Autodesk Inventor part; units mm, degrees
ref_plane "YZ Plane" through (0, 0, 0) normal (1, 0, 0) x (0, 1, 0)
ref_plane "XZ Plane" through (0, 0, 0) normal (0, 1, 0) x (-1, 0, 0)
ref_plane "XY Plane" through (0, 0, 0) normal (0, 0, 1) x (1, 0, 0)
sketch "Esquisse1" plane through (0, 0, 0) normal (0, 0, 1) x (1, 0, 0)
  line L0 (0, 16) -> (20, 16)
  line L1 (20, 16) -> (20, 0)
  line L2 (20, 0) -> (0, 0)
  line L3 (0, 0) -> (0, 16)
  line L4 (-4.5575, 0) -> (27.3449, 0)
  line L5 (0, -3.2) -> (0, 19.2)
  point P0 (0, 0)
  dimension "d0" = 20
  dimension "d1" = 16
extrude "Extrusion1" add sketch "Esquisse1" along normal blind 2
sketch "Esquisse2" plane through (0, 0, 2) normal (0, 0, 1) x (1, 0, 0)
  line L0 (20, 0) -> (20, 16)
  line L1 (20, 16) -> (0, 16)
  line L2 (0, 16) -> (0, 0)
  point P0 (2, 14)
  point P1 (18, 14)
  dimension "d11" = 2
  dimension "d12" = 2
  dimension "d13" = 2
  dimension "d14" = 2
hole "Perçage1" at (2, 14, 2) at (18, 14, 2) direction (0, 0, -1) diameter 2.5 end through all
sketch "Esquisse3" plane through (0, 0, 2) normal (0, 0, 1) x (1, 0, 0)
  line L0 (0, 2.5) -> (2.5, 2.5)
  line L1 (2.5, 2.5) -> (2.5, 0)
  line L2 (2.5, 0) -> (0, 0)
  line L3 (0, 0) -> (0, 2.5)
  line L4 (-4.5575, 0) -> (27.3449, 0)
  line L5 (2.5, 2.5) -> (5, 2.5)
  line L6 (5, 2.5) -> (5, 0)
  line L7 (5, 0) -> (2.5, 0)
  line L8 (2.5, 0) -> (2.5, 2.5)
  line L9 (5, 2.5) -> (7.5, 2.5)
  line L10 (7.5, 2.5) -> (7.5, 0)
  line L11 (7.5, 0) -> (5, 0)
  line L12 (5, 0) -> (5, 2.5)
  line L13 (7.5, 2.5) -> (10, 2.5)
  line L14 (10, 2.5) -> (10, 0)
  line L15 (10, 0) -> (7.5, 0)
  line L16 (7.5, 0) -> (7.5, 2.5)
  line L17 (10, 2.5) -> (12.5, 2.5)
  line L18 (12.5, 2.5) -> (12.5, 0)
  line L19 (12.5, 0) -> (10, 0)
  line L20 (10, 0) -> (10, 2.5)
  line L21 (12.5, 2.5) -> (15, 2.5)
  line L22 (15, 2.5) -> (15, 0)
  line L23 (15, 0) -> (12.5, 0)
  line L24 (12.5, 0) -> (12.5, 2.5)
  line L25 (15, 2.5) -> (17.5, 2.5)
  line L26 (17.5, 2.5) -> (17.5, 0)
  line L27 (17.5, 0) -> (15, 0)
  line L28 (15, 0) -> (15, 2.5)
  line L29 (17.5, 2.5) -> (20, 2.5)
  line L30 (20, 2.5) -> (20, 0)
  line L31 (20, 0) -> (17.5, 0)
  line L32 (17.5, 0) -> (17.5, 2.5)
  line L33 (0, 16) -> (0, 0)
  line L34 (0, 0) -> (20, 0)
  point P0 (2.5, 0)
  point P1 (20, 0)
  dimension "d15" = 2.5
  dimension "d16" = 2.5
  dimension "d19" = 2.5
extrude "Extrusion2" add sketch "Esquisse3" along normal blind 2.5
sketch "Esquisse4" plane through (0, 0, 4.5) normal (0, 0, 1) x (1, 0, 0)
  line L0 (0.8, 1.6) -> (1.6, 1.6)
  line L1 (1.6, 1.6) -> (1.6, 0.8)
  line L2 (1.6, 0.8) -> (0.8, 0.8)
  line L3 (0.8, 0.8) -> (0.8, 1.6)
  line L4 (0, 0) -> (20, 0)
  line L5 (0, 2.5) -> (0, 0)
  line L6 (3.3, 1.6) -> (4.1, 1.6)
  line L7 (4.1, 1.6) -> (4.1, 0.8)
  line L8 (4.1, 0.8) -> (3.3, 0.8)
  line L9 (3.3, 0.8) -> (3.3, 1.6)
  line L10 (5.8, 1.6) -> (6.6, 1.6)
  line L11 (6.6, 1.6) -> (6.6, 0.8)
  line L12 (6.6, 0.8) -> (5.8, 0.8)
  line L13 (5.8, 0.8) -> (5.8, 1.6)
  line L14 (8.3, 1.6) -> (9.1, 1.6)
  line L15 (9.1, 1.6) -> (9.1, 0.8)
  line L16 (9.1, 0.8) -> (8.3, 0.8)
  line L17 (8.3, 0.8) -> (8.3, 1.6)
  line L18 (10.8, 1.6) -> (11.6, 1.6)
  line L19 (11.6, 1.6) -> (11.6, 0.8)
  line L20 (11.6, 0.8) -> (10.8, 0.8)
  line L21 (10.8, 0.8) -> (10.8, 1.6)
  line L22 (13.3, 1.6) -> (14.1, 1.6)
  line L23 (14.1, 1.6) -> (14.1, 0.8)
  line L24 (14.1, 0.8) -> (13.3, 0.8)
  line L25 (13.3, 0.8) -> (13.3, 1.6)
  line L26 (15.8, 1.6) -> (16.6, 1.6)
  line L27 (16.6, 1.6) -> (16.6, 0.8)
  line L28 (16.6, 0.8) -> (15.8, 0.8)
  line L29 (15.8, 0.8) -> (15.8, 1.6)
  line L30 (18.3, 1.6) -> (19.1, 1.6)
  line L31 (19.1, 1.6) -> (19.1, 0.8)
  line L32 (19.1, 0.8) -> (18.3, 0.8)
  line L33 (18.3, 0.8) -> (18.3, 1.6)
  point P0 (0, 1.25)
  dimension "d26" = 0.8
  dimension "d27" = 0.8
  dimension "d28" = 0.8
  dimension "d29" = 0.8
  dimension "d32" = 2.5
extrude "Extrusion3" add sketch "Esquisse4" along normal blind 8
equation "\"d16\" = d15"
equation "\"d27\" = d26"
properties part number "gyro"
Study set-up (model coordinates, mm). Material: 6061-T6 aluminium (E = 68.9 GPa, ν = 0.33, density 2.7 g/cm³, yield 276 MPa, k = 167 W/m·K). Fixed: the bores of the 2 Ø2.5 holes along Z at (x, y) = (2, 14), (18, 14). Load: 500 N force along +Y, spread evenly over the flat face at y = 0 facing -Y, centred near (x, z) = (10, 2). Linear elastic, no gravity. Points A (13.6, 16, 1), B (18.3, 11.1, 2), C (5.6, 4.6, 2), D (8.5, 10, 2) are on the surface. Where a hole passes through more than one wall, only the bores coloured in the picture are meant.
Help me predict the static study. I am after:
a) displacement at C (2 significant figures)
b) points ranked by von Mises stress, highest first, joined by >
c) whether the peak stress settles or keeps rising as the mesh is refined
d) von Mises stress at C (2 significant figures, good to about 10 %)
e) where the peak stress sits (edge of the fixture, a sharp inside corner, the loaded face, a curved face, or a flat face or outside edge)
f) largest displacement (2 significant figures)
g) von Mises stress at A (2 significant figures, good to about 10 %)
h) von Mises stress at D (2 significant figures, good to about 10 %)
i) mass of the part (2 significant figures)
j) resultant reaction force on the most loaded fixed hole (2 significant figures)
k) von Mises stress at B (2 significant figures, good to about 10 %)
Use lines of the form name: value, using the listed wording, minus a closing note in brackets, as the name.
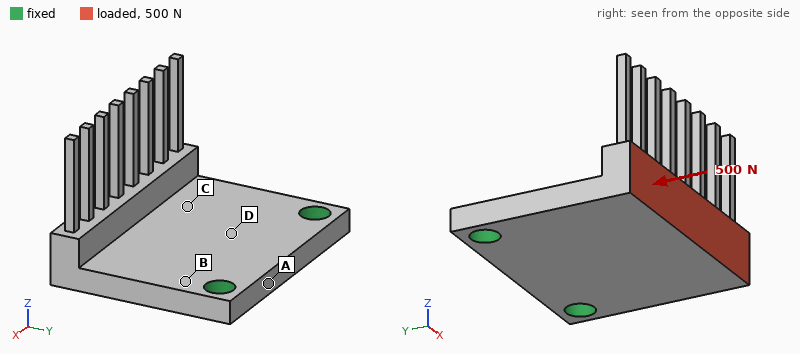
displacement at C: 0.034 mm
points ranked by von Mises stress, highest first, joined by >: B > C > D > A
whether the peak stress settles or keeps rising as the mesh is refined: keeps rising
von Mises stress at C: 54 MPa
where the peak stress sits: edge of the fixture
largest displacement: 0.12 mm
von Mises stress at A: 23 MPa
von Mises stress at D: 40 MPa
mass of the part: 2.1 g
resultant reaction force on the most loaded fixed hole: 260 N
von Mises stress at B: 85 MPa
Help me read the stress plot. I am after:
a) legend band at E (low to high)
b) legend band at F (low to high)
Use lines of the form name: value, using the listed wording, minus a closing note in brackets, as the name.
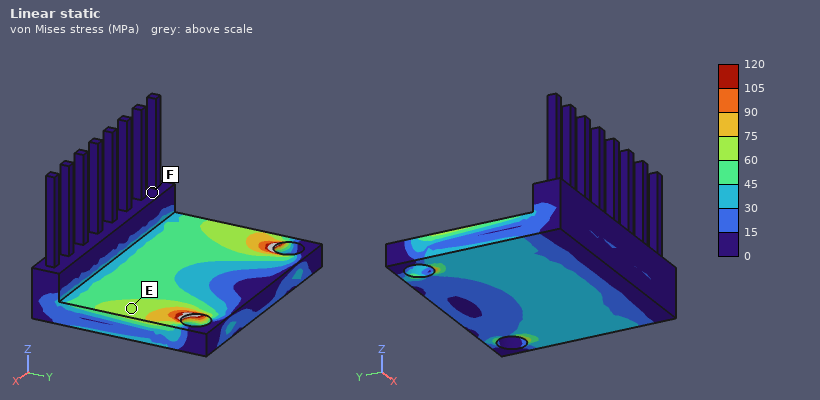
legend band at E: 60 to 75 MPa
legend band at F: 0 to 15 MPa
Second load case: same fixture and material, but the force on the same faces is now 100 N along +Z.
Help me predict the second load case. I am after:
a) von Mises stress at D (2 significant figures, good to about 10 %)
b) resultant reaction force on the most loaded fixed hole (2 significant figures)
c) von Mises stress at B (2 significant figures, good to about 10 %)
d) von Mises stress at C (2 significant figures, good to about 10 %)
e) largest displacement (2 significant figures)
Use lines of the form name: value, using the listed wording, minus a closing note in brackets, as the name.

von Mises stress at D: 52 MPa
resultant reaction force on the most loaded fixed hole: 50 N
von Mises stress at B: 120 MPa
von Mises stress at C: 34 MPa
largest displacement: 0.16 mm
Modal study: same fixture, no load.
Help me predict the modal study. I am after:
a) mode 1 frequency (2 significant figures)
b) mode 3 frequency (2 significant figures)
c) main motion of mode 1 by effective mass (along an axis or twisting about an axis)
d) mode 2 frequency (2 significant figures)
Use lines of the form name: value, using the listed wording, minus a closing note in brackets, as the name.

mode 1 frequency: 5300 Hz
mode 3 frequency: 9500 Hz
main motion of mode 1 by effective mass: along Z
mode 2 frequency: 8800 Hz
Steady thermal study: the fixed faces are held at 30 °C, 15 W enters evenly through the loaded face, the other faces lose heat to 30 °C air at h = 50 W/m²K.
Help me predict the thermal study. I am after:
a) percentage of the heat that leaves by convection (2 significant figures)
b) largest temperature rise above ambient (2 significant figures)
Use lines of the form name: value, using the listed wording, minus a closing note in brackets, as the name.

percentage of the heat that leaves by convection: 6.4 %
largest temperature rise above ambient: 32 K
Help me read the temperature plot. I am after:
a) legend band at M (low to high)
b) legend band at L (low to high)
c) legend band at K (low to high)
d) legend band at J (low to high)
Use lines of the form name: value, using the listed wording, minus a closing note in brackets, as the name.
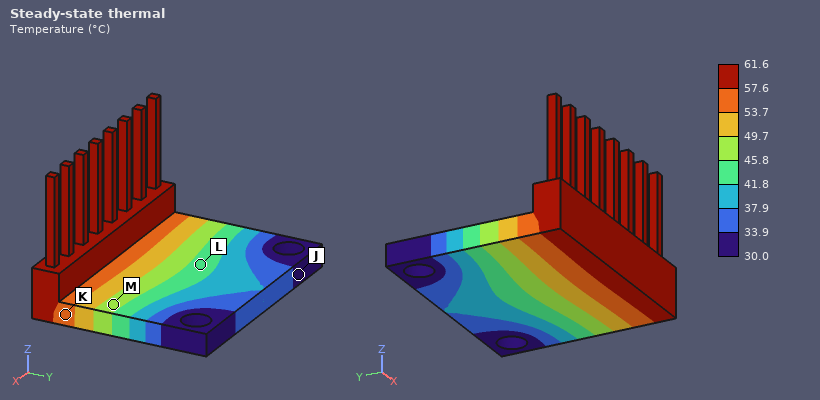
legend band at M: 45.8 to 49.7 °C
legend band at L: 41.8 to 45.8 °C
legend band at K: 53.7 to 57.6 °C
legend band at J: 30.0 to 33.9 °C
